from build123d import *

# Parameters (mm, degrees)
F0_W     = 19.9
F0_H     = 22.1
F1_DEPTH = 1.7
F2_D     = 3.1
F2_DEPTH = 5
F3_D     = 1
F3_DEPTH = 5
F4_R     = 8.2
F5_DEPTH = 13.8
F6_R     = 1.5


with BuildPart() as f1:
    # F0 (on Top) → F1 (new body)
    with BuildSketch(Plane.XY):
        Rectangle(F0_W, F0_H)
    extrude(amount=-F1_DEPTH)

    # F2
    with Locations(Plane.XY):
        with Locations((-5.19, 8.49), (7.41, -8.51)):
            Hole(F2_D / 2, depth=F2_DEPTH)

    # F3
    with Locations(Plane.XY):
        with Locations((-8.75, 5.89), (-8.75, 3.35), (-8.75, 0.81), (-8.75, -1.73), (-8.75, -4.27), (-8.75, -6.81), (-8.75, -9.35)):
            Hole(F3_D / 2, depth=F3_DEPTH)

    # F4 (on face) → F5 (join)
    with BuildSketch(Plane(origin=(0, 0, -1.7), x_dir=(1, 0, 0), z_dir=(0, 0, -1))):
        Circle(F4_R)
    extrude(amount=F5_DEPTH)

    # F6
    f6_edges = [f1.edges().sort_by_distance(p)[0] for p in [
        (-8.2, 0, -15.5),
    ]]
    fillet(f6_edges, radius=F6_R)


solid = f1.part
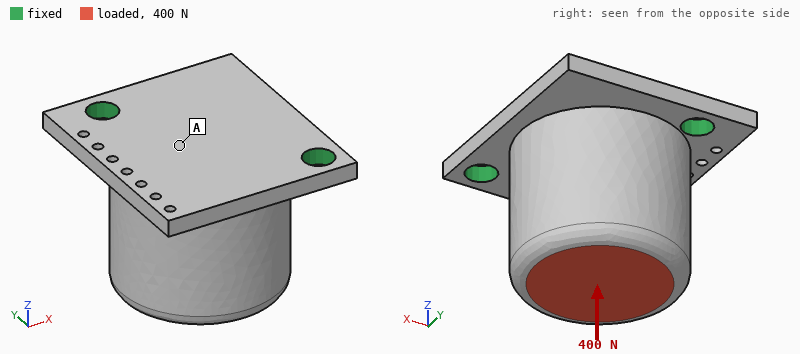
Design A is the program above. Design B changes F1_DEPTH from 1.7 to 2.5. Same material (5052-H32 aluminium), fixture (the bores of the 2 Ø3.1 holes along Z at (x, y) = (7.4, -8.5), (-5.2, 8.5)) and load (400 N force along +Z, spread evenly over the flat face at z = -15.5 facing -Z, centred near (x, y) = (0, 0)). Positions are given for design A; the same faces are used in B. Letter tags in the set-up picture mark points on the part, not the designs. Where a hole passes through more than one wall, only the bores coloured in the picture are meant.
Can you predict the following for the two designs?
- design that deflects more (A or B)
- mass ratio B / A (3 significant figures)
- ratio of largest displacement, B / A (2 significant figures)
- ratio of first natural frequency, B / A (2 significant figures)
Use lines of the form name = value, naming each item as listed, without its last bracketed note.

design that deflects more = A
mass ratio B / A = 1.05
ratio of largest displacement, B / A = 0.54
ratio of first natural frequency, B / A = 1.5
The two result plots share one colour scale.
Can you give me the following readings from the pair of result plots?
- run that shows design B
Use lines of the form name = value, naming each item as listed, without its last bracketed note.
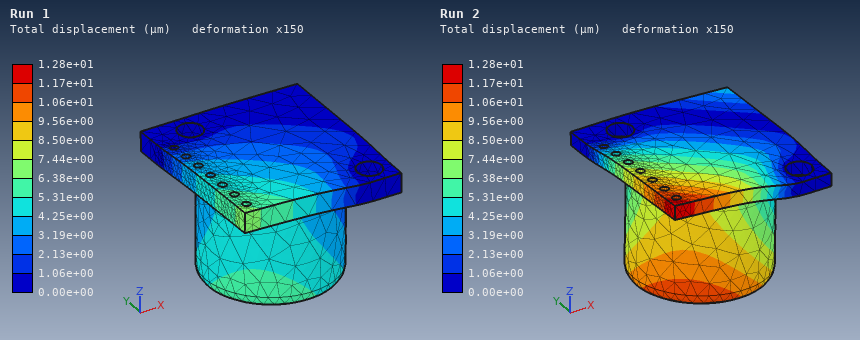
run that shows design B = Run 1
